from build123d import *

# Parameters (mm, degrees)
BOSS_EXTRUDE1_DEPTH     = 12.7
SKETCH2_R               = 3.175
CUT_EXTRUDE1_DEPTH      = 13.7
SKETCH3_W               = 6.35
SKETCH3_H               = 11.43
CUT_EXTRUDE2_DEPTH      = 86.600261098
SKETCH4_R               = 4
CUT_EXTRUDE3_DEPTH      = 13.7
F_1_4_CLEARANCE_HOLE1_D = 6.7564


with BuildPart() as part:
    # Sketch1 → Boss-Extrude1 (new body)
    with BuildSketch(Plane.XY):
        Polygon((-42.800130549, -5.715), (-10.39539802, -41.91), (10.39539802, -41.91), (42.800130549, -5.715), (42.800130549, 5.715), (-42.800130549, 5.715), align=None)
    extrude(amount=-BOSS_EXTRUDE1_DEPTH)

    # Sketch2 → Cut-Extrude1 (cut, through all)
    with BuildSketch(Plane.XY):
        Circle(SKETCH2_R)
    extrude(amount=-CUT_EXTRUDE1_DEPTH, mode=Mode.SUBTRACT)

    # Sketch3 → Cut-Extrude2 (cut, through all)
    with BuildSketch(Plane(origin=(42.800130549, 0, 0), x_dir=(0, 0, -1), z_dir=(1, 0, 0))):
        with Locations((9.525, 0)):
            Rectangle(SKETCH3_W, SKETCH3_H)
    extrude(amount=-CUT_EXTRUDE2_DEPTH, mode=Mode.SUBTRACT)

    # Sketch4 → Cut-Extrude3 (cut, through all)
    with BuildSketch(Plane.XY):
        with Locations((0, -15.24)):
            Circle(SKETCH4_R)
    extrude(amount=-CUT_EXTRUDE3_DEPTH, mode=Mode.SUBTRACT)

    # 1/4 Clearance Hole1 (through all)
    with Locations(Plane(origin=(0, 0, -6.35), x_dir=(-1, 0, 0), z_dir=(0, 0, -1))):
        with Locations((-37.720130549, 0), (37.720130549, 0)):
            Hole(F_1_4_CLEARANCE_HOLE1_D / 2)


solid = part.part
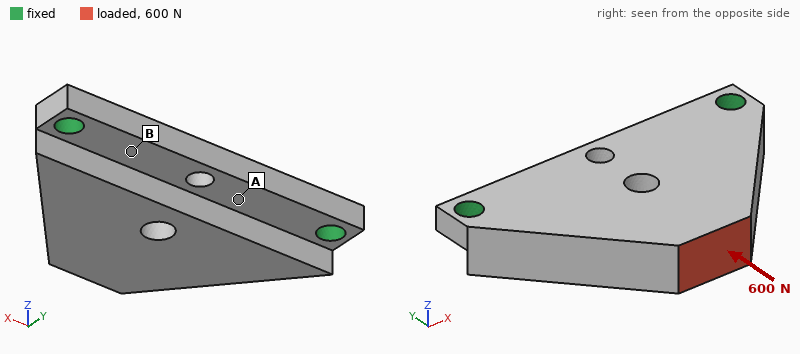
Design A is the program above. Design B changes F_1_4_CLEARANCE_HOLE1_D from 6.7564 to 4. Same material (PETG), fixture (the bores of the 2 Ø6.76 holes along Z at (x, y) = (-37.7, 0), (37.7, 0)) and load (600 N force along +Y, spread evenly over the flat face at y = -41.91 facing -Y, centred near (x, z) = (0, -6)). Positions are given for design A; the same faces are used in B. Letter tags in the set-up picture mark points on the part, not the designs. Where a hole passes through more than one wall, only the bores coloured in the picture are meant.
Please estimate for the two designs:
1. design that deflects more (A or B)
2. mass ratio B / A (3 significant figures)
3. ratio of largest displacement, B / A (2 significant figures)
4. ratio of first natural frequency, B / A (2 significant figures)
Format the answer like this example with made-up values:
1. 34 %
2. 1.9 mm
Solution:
1. B
2. 1.01
3. 1.3
4. 0.87
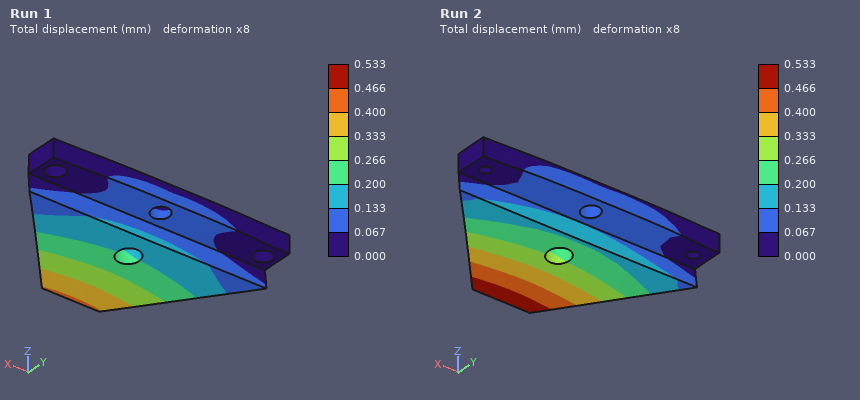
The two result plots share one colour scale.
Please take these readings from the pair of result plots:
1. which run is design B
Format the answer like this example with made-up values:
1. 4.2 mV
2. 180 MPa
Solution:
1. Run 2
